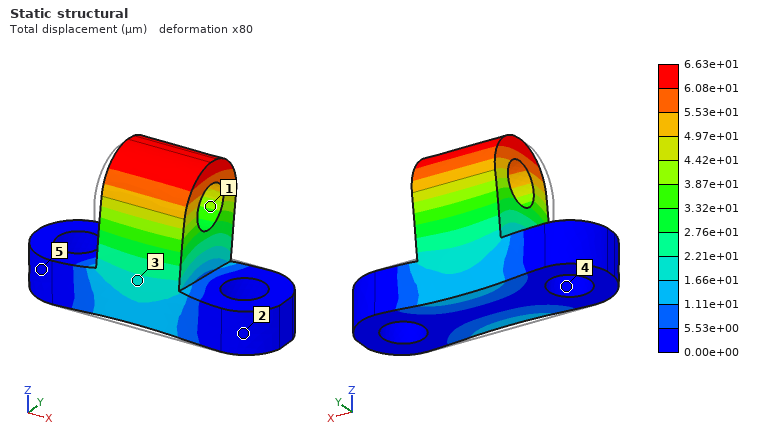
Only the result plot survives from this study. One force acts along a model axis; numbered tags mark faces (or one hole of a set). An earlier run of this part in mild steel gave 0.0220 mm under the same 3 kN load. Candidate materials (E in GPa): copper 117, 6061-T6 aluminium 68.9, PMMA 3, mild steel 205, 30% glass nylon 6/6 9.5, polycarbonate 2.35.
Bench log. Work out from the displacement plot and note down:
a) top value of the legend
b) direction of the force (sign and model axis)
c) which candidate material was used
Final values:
6.63e+01 µm
+Y
6061-T6 aluminium
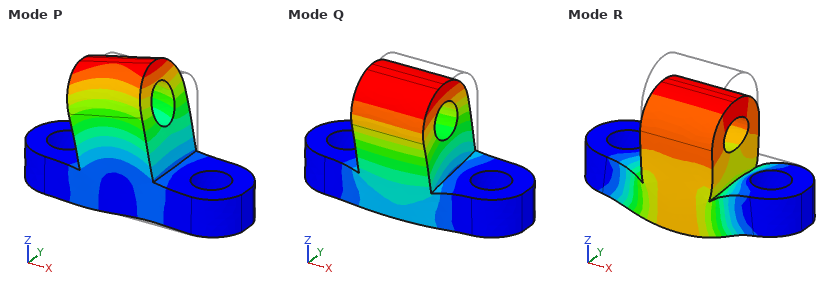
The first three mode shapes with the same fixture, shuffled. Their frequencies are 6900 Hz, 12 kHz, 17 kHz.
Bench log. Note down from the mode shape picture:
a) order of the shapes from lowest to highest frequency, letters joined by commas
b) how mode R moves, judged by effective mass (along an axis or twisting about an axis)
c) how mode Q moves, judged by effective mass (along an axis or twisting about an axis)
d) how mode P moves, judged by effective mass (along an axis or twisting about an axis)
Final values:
Q, P, R
along Z
along Y
along X
